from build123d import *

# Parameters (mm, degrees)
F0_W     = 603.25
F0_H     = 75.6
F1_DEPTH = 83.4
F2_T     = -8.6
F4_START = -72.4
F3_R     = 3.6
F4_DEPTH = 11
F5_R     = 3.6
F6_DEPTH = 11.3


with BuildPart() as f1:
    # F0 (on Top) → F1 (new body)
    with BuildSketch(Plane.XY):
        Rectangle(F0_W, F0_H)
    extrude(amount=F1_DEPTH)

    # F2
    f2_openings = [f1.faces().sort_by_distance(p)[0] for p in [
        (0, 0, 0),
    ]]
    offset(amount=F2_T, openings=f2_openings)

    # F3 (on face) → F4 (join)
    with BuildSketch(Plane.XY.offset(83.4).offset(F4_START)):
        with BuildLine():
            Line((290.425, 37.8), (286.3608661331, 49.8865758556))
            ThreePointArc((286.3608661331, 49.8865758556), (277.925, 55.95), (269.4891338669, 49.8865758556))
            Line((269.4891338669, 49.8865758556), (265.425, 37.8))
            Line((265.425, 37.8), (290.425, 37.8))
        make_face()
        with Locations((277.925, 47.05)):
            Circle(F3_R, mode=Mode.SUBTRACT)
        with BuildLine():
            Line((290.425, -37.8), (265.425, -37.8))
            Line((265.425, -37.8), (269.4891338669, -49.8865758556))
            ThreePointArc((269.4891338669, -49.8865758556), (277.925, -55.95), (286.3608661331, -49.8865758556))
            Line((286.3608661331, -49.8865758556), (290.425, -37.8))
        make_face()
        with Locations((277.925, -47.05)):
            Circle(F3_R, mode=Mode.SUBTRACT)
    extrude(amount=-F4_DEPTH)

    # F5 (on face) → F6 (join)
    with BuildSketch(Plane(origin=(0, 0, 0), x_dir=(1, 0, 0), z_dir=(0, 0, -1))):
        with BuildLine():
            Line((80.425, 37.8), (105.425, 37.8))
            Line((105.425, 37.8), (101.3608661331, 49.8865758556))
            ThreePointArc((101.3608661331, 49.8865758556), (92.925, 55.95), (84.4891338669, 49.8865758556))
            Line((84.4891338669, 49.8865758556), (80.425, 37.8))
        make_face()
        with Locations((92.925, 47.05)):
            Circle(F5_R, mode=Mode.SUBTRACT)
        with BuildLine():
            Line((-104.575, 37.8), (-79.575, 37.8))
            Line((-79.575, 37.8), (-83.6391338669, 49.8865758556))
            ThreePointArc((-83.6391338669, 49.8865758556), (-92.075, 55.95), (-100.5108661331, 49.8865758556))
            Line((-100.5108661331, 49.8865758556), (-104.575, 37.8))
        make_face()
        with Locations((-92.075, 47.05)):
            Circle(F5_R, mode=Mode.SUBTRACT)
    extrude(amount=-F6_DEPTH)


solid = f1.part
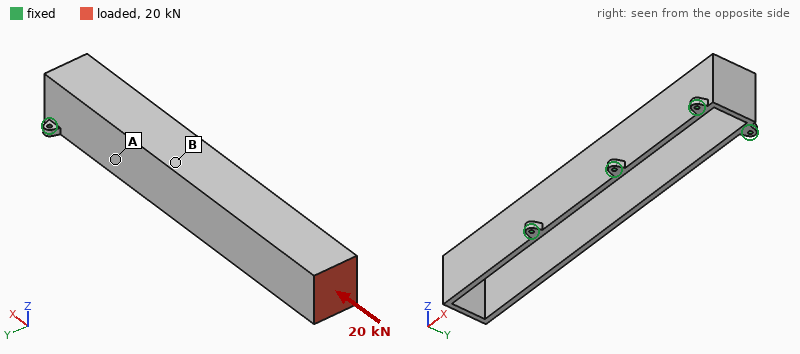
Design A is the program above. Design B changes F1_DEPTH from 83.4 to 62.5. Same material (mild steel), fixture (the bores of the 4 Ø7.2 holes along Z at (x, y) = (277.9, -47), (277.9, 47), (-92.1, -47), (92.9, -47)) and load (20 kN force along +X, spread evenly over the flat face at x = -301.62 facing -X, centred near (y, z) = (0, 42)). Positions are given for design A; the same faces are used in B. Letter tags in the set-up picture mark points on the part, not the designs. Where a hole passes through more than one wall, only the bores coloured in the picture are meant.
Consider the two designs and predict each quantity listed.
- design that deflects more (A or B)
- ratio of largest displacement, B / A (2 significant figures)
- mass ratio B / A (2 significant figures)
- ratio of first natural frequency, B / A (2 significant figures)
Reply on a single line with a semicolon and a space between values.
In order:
B; 1.3; 0.81; 1.1
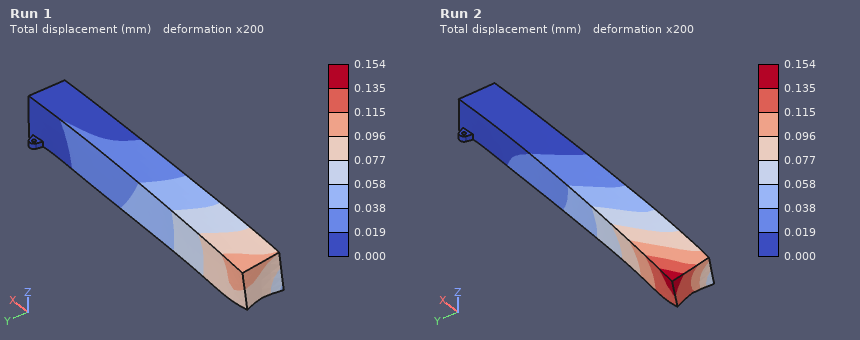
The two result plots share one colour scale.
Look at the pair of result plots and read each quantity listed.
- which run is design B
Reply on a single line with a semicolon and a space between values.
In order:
Run 2
